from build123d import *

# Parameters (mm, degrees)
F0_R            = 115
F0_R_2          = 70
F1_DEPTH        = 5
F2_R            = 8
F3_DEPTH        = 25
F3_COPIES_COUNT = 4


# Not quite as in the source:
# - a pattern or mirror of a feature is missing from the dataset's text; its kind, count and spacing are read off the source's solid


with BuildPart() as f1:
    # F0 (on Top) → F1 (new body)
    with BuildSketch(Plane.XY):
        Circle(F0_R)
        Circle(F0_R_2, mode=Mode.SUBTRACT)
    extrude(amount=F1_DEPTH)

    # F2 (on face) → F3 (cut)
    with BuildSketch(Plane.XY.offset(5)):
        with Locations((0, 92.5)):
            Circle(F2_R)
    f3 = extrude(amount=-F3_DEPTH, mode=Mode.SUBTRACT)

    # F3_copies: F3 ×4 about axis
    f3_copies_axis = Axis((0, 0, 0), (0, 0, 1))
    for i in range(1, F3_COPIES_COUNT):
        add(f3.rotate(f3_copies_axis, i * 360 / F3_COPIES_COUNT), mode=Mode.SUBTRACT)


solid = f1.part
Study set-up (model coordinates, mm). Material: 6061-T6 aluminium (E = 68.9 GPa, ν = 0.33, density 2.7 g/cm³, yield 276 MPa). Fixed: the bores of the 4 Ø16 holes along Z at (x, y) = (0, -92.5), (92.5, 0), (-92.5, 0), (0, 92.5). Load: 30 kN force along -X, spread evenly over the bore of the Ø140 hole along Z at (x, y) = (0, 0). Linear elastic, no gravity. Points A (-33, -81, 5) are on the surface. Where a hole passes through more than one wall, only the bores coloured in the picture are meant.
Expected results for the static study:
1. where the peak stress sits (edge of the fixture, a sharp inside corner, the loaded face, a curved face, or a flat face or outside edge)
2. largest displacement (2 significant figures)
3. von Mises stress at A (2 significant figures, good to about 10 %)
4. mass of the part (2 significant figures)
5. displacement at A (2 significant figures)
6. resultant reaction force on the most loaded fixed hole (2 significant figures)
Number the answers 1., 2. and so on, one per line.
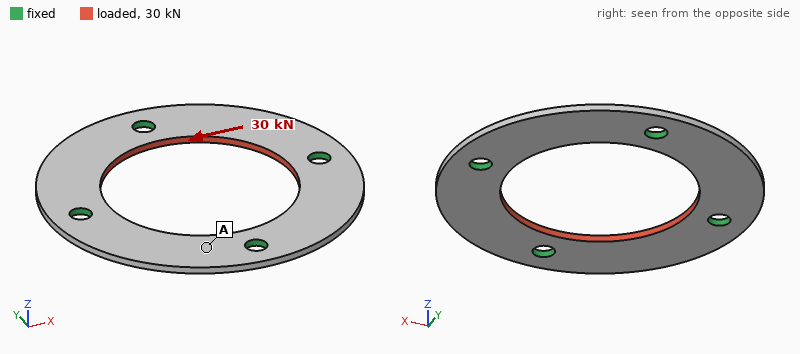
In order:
1. edge of the fixture
2. 31 µm
3. 18 MPa
4. 340 g
5. 17 µm
6. 9.0 kN
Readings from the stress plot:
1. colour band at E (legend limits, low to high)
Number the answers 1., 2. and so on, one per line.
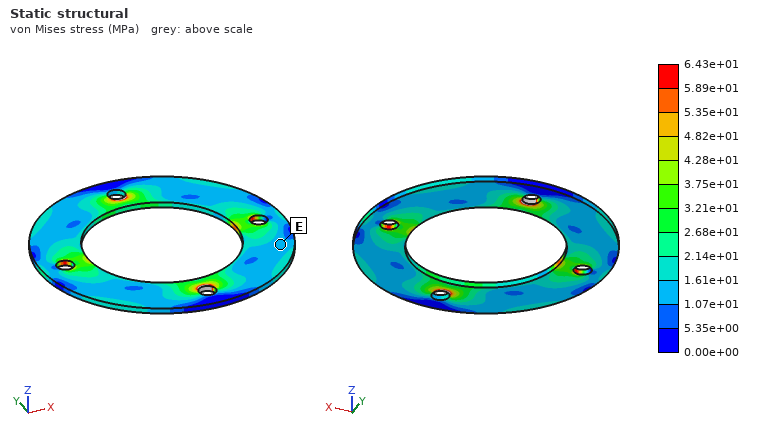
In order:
1. 1.07e+01 to 1.61e+01 MPa
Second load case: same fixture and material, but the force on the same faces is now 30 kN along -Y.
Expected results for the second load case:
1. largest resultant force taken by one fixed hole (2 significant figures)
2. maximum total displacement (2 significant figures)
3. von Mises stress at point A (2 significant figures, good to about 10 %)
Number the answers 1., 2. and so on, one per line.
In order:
1. 9.0 kN
2. 31 µm
3. 19 MPa
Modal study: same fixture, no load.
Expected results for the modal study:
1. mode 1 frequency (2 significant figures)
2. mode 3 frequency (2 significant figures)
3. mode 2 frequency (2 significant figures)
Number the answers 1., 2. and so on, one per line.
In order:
1. 1200 Hz
2. 1200 Hz
3. 1200 Hz
